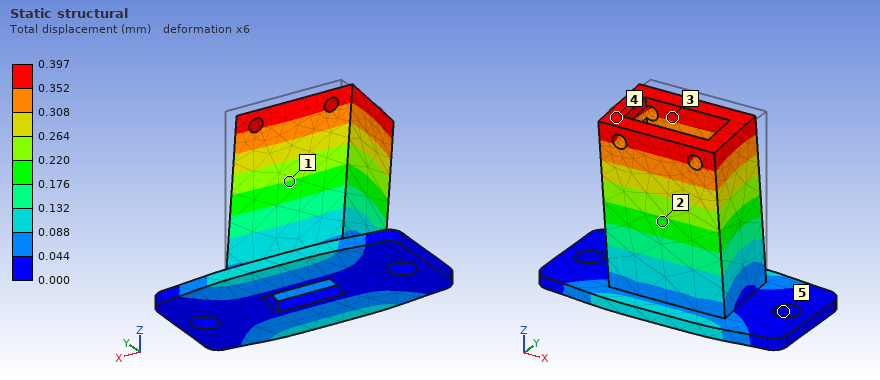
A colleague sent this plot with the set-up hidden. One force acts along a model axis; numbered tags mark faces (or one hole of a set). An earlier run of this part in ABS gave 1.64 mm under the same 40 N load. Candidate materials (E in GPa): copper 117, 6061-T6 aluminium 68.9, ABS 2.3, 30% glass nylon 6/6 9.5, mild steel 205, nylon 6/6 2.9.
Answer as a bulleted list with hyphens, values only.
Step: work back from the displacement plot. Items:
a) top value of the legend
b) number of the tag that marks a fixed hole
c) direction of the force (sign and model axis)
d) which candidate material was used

- 0.397 mm
- 5
- -Y
- 30% glass nylon 6/6
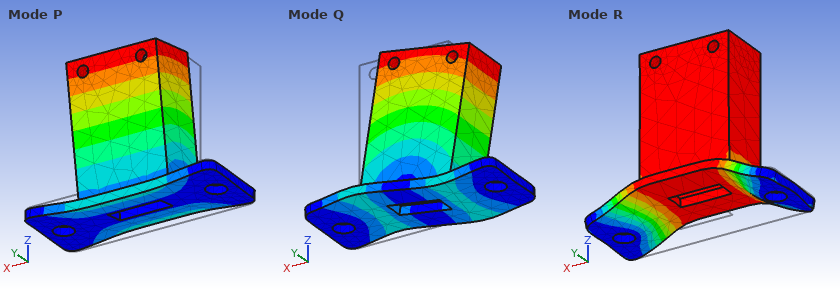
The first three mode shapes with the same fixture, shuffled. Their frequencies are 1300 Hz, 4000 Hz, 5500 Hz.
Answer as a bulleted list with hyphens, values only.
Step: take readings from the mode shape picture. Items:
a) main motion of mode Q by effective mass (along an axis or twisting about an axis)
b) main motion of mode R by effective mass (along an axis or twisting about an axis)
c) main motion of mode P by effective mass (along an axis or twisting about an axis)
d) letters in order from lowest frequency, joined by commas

- along X
- along Z
- along Y
- P, Q, R
